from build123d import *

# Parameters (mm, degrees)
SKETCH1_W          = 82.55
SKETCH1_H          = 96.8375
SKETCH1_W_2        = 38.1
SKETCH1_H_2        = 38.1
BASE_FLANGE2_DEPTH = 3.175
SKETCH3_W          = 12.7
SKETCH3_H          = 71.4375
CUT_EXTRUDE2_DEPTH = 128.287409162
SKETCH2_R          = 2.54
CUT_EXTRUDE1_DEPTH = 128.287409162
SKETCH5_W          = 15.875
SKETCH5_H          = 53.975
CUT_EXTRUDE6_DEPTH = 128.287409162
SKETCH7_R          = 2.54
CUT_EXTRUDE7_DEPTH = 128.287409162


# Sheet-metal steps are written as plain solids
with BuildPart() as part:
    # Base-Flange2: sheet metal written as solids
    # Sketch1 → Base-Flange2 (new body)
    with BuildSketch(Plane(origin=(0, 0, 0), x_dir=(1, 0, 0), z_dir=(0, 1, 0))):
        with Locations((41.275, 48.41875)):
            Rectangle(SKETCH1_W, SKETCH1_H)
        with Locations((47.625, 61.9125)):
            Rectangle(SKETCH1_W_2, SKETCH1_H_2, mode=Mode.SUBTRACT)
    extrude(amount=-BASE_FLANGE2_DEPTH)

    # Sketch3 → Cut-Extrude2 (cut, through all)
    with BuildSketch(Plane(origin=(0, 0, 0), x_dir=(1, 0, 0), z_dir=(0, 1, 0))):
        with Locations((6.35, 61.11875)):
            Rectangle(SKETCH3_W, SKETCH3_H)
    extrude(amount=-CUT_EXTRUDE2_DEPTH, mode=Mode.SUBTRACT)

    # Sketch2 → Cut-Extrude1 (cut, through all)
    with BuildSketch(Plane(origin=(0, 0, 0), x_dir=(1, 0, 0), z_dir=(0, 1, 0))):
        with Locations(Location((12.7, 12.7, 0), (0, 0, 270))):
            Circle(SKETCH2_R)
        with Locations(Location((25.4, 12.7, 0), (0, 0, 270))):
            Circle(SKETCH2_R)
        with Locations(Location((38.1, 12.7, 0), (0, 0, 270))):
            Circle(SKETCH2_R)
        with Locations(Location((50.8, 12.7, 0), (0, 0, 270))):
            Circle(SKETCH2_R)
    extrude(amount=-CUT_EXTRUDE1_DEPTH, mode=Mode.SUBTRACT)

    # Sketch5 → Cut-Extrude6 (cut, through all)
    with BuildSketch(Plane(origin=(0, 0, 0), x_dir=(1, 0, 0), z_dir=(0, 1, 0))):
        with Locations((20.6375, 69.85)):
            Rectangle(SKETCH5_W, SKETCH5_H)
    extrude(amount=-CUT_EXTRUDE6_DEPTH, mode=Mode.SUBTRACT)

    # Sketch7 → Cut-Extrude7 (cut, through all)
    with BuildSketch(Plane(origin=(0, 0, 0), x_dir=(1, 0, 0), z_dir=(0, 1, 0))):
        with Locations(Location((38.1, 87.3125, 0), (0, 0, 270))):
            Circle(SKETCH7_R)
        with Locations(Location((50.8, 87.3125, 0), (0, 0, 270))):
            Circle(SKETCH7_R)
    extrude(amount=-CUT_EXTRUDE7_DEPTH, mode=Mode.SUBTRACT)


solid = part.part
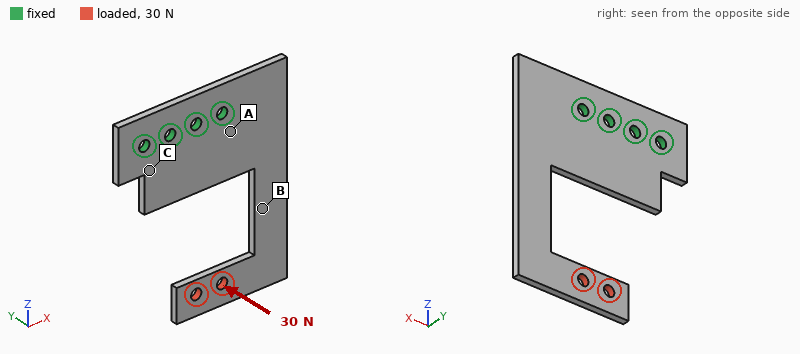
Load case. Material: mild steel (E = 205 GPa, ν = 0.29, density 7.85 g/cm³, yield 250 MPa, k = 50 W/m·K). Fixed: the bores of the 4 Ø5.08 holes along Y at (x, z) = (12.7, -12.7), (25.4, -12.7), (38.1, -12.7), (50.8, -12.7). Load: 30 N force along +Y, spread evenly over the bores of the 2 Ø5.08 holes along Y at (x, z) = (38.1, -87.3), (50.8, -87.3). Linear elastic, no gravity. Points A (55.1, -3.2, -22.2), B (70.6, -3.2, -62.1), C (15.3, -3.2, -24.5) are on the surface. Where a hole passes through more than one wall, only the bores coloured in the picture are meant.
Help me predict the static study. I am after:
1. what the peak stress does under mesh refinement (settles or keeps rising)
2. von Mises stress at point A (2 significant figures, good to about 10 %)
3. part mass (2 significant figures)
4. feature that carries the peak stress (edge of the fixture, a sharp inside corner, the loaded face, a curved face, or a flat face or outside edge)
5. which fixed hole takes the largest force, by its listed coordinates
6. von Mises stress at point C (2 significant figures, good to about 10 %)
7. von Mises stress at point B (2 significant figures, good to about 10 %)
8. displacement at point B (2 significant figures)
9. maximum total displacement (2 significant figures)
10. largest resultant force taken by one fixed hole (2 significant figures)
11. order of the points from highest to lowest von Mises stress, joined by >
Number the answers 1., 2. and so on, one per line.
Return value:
1. keeps rising
2. 23 MPa
3. 120 g
4. a sharp inside corner
5. (38.1, -12.7)
6. 9.2 MPa
7. 45 MPa
8. 0.13 mm
9. 0.55 mm
10. 25 N
11. B > A > C
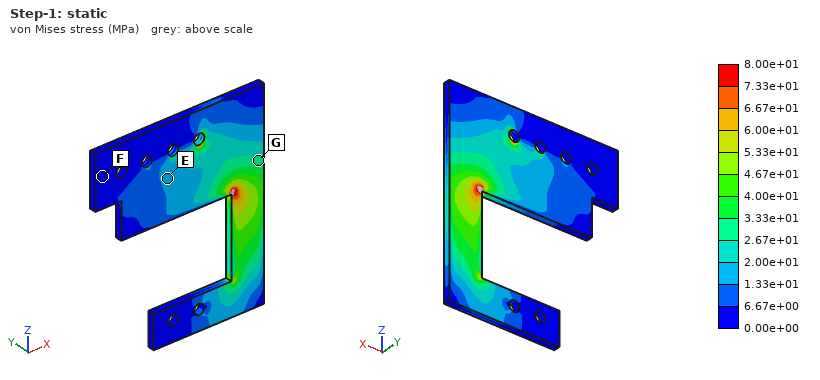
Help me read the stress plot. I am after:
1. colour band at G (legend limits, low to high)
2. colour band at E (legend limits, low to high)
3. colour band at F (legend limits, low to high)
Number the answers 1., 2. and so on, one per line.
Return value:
1. 2.67e+01 to 3.33e+01 MPa
2. 1.33e+01 to 2.00e+01 MPa
3. 0.00e+00 to 6.67e+00 MPa
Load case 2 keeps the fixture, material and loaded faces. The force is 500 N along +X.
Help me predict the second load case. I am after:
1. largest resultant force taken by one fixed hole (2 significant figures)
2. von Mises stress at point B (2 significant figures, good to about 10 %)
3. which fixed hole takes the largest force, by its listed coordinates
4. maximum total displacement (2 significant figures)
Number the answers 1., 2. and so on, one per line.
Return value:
1. 1.1 kN
2. 52 MPa
3. (50.8, -12.7)
4. 0.24 mm
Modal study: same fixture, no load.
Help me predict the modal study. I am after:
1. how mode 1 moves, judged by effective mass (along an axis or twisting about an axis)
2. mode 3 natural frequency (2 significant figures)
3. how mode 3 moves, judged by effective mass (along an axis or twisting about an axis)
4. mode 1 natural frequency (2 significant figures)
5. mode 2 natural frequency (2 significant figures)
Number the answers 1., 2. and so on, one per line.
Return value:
1. along Y
2. 1600 Hz
3. along X
4. 300 Hz
5. 760 Hz
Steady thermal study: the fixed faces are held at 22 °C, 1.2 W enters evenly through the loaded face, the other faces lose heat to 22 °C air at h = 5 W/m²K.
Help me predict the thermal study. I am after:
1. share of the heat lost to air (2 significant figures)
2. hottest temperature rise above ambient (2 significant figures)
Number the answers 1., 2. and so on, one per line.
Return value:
1. 35 %
2. 34 K
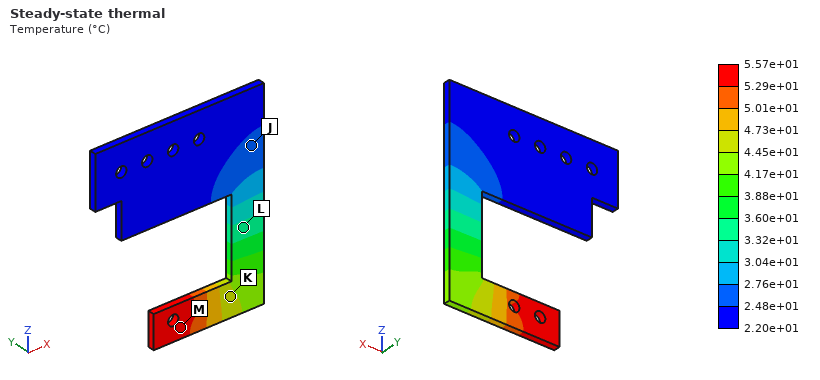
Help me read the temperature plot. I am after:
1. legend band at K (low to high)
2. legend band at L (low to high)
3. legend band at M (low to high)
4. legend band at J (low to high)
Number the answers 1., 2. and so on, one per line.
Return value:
1. 4.45e+01 to 4.73e+01 °C
2. 3.32e+01 to 3.60e+01 °C
3. 5.29e+01 to 5.57e+01 °C
4. 2.48e+01 to 2.76e+01 °C
